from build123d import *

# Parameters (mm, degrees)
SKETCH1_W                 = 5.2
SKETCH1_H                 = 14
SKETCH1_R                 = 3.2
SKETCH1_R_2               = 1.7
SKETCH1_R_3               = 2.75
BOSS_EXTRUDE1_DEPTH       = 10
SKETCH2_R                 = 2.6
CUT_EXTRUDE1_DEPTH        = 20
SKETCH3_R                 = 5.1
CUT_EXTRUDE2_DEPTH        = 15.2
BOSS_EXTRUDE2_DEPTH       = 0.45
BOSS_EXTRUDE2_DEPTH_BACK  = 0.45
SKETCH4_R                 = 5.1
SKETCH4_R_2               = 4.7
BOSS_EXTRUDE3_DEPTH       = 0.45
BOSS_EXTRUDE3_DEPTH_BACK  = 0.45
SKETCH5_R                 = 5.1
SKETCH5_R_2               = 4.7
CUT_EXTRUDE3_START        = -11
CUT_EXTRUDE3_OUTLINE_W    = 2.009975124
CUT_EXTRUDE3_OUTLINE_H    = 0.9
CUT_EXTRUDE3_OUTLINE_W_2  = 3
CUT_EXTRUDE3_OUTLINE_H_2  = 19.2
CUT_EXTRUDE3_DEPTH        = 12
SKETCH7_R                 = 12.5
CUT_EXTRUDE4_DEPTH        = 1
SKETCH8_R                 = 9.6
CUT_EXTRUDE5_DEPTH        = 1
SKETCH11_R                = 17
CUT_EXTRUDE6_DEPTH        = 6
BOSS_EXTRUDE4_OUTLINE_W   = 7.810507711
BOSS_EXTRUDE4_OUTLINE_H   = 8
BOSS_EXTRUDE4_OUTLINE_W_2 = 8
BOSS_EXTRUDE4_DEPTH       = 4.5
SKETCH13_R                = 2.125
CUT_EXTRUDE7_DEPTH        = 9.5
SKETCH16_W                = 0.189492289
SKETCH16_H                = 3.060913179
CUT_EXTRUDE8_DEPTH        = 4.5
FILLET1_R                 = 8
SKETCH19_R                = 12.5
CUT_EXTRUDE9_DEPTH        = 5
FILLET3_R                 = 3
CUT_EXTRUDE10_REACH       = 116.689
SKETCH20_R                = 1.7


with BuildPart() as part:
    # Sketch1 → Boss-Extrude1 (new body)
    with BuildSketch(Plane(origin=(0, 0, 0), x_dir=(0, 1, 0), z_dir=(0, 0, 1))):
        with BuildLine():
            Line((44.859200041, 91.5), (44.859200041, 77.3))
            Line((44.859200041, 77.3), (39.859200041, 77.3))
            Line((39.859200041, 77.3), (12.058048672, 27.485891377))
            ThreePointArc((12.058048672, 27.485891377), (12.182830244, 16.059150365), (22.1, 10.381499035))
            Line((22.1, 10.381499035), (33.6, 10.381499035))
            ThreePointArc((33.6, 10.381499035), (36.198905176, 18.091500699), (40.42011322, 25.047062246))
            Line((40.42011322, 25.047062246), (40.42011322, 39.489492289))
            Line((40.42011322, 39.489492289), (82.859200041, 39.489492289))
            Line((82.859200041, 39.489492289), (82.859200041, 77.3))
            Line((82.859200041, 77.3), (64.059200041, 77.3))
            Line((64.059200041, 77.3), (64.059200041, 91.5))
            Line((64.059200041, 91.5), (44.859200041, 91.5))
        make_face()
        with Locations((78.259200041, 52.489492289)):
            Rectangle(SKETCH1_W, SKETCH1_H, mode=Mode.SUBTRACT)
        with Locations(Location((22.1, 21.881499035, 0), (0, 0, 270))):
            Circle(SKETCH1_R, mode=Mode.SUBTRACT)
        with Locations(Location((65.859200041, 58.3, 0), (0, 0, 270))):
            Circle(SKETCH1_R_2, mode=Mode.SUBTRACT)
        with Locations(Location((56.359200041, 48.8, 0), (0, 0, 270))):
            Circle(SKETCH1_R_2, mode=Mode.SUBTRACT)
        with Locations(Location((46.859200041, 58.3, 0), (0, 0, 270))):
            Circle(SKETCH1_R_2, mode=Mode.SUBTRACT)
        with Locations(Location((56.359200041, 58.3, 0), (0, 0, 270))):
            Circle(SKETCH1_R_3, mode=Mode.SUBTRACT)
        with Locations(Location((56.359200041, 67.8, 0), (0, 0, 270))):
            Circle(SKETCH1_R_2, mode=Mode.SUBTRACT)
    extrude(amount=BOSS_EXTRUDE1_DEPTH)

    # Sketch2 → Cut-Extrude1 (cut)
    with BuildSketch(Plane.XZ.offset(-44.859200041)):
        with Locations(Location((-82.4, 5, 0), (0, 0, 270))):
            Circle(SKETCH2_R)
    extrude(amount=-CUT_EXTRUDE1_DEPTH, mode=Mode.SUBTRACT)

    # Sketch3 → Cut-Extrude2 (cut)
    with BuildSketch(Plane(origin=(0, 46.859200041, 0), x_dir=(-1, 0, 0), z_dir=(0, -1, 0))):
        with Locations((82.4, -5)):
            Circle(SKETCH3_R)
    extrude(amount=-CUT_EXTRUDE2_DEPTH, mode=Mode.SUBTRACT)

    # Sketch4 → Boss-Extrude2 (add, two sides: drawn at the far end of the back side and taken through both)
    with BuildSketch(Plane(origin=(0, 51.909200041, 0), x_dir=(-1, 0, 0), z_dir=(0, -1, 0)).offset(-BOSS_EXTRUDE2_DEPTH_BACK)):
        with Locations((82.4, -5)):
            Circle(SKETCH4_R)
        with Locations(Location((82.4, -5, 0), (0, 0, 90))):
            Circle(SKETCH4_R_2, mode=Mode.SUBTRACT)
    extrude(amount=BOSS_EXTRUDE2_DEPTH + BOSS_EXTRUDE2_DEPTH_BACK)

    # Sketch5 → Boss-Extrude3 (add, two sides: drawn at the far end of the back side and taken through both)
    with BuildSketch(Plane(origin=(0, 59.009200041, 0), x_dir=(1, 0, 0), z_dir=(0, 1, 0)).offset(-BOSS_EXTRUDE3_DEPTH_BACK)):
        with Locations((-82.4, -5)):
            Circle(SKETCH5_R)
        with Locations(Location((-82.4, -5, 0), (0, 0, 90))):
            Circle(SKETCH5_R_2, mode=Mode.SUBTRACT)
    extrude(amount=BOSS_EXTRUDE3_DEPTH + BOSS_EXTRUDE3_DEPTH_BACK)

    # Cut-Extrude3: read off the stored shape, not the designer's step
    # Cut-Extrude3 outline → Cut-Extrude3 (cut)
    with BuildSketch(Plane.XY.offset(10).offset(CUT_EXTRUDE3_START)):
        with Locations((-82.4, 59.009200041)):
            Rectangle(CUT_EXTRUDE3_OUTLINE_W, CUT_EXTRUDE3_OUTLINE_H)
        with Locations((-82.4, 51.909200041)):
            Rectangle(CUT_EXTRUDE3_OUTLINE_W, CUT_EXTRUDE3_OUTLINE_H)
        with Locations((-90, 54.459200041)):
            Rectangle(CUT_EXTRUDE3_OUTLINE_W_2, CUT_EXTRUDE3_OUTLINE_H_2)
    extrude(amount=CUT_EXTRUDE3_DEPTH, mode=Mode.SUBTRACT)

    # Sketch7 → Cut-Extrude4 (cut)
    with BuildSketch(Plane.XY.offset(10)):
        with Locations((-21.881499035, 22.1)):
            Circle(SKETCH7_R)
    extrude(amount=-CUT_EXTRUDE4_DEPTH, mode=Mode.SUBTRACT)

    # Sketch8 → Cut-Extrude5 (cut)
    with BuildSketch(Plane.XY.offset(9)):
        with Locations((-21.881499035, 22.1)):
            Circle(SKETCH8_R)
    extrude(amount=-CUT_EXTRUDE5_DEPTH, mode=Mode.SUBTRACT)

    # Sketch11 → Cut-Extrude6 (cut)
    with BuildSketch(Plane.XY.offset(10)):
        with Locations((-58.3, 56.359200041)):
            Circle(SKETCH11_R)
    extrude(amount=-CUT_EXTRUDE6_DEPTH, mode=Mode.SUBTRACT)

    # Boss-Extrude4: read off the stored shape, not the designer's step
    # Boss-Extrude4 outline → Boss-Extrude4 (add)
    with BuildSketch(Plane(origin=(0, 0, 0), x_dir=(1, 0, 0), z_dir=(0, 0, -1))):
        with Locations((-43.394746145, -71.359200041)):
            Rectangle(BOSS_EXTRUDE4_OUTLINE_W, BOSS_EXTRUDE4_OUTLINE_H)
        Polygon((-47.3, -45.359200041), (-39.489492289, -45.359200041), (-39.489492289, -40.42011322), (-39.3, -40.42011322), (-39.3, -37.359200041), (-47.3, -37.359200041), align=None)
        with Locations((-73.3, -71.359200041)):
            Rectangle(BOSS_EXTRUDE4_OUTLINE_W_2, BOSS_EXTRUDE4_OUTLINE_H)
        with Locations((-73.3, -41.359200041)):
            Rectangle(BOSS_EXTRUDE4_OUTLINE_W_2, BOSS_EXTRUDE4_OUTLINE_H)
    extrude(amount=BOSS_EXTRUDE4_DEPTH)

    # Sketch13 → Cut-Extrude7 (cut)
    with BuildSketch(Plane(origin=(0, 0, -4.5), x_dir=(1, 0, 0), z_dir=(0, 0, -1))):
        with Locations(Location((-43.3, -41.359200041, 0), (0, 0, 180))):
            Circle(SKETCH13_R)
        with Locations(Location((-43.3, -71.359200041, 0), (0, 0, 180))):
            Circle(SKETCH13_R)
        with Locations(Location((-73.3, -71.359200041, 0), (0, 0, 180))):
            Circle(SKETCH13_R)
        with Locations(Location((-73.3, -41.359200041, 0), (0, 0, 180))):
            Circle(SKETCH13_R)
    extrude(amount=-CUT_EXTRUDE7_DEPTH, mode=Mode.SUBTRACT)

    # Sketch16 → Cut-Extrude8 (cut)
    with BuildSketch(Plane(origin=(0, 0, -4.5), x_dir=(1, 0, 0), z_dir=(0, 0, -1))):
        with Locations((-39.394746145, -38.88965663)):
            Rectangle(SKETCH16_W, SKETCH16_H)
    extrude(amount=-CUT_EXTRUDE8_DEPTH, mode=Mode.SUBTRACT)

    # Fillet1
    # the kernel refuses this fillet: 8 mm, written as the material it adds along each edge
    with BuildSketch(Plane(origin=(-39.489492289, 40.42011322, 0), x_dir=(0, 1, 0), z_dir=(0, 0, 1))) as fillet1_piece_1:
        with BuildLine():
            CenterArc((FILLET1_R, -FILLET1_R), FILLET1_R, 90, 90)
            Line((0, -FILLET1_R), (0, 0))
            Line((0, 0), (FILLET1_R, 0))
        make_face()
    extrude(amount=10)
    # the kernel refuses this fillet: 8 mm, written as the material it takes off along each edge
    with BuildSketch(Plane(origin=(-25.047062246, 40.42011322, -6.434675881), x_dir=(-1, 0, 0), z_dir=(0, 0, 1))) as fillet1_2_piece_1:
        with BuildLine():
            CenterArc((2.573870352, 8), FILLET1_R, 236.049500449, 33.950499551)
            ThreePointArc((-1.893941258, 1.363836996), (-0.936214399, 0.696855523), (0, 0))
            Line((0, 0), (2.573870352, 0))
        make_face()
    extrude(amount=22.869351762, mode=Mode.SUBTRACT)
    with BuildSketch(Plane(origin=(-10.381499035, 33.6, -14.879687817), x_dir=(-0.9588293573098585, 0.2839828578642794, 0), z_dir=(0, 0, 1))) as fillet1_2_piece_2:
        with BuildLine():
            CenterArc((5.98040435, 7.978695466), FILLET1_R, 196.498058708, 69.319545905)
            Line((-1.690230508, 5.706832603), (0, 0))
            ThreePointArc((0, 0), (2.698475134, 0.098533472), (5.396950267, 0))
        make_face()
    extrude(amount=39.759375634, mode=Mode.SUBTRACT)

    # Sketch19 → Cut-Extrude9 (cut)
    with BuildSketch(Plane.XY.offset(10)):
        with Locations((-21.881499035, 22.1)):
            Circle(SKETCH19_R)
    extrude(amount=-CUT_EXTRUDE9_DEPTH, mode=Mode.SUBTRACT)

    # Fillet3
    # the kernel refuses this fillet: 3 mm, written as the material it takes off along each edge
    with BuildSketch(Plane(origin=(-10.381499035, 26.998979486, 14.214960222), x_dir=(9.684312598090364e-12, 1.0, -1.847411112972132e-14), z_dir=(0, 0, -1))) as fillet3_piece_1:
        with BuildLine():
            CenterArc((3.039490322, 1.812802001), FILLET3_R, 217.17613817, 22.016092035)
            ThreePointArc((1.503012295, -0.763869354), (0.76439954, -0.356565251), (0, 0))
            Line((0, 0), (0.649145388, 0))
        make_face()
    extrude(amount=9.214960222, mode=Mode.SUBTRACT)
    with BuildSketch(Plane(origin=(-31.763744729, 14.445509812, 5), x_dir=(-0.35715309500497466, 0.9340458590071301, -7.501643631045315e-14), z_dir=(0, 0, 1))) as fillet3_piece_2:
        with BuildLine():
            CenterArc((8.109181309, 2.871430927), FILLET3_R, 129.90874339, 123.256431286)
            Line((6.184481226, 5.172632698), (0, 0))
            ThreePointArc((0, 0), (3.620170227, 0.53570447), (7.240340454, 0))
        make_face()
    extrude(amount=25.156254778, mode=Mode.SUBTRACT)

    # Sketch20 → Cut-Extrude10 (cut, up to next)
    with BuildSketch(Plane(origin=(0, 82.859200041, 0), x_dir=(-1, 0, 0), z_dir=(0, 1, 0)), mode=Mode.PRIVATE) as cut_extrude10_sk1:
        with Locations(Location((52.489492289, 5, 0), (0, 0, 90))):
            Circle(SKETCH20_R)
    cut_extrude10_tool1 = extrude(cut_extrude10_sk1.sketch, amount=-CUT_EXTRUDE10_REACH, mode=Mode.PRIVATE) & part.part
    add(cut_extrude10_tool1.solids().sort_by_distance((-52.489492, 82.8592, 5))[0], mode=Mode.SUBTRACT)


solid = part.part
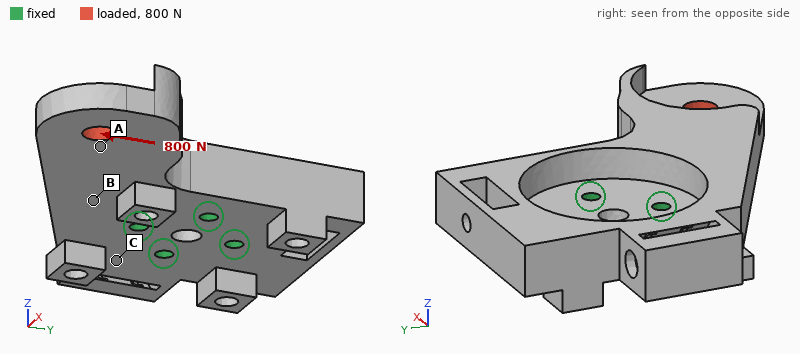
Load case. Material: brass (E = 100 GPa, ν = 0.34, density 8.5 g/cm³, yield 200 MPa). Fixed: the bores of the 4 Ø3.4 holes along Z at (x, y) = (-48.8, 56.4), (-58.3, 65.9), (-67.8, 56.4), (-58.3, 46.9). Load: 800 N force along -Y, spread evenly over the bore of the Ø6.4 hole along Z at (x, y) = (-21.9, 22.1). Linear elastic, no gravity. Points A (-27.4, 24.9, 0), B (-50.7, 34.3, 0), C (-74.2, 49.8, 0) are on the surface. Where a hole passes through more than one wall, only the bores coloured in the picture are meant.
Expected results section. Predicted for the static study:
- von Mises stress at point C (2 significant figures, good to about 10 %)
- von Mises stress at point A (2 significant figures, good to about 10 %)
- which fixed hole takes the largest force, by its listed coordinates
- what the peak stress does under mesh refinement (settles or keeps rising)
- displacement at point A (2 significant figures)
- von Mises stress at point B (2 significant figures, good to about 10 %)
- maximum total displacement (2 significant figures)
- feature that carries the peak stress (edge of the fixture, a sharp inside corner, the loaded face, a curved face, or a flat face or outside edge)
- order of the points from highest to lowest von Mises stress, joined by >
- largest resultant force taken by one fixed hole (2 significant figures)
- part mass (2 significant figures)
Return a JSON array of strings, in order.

["4.9 MPa", "19 MPa", "(-48.8, 56.4)", "keeps rising", "25 µm", "12 MPa", "42 µm", "edge of the fixture", "A > B > C", "1.3 kN", "170 g"]
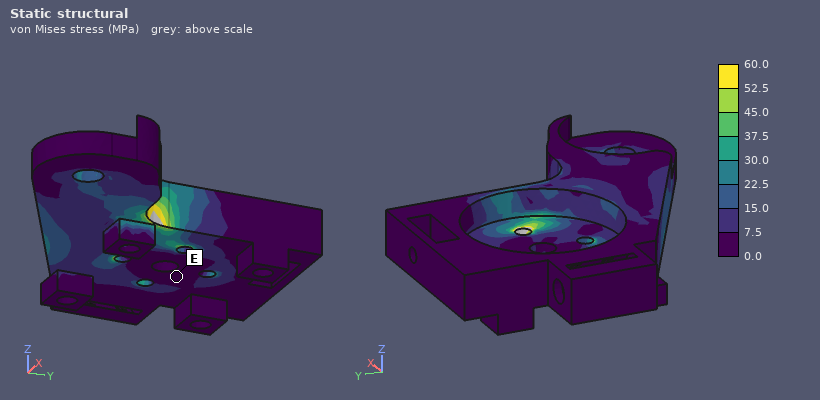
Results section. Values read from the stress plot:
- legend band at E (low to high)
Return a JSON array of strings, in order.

["0.0 to 7.5 MPa"]
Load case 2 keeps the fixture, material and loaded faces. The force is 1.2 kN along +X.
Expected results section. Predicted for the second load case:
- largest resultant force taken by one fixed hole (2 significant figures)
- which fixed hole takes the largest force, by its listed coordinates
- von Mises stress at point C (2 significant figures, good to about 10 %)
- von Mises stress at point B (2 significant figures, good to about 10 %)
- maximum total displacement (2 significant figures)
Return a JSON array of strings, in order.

["1.5 kN", "(-58.3, 46.9)", "8.2 MPa", "23 MPa", "48 µm"]
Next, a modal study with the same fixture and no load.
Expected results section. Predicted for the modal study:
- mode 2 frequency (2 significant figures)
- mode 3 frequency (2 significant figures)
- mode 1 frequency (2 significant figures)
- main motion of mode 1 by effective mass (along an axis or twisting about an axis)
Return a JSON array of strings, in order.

["4200 Hz", "4500 Hz", "1400 Hz", "along Z"]
